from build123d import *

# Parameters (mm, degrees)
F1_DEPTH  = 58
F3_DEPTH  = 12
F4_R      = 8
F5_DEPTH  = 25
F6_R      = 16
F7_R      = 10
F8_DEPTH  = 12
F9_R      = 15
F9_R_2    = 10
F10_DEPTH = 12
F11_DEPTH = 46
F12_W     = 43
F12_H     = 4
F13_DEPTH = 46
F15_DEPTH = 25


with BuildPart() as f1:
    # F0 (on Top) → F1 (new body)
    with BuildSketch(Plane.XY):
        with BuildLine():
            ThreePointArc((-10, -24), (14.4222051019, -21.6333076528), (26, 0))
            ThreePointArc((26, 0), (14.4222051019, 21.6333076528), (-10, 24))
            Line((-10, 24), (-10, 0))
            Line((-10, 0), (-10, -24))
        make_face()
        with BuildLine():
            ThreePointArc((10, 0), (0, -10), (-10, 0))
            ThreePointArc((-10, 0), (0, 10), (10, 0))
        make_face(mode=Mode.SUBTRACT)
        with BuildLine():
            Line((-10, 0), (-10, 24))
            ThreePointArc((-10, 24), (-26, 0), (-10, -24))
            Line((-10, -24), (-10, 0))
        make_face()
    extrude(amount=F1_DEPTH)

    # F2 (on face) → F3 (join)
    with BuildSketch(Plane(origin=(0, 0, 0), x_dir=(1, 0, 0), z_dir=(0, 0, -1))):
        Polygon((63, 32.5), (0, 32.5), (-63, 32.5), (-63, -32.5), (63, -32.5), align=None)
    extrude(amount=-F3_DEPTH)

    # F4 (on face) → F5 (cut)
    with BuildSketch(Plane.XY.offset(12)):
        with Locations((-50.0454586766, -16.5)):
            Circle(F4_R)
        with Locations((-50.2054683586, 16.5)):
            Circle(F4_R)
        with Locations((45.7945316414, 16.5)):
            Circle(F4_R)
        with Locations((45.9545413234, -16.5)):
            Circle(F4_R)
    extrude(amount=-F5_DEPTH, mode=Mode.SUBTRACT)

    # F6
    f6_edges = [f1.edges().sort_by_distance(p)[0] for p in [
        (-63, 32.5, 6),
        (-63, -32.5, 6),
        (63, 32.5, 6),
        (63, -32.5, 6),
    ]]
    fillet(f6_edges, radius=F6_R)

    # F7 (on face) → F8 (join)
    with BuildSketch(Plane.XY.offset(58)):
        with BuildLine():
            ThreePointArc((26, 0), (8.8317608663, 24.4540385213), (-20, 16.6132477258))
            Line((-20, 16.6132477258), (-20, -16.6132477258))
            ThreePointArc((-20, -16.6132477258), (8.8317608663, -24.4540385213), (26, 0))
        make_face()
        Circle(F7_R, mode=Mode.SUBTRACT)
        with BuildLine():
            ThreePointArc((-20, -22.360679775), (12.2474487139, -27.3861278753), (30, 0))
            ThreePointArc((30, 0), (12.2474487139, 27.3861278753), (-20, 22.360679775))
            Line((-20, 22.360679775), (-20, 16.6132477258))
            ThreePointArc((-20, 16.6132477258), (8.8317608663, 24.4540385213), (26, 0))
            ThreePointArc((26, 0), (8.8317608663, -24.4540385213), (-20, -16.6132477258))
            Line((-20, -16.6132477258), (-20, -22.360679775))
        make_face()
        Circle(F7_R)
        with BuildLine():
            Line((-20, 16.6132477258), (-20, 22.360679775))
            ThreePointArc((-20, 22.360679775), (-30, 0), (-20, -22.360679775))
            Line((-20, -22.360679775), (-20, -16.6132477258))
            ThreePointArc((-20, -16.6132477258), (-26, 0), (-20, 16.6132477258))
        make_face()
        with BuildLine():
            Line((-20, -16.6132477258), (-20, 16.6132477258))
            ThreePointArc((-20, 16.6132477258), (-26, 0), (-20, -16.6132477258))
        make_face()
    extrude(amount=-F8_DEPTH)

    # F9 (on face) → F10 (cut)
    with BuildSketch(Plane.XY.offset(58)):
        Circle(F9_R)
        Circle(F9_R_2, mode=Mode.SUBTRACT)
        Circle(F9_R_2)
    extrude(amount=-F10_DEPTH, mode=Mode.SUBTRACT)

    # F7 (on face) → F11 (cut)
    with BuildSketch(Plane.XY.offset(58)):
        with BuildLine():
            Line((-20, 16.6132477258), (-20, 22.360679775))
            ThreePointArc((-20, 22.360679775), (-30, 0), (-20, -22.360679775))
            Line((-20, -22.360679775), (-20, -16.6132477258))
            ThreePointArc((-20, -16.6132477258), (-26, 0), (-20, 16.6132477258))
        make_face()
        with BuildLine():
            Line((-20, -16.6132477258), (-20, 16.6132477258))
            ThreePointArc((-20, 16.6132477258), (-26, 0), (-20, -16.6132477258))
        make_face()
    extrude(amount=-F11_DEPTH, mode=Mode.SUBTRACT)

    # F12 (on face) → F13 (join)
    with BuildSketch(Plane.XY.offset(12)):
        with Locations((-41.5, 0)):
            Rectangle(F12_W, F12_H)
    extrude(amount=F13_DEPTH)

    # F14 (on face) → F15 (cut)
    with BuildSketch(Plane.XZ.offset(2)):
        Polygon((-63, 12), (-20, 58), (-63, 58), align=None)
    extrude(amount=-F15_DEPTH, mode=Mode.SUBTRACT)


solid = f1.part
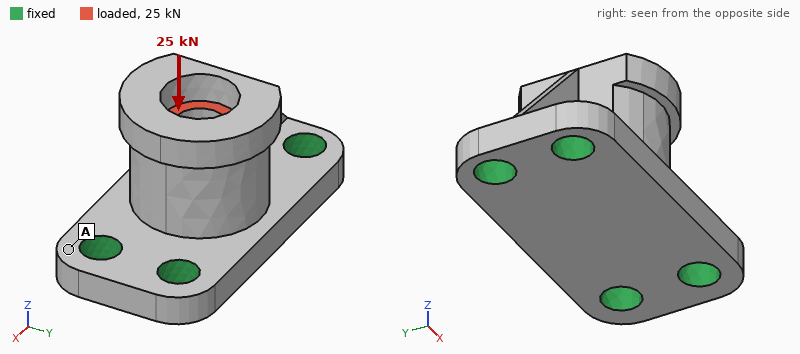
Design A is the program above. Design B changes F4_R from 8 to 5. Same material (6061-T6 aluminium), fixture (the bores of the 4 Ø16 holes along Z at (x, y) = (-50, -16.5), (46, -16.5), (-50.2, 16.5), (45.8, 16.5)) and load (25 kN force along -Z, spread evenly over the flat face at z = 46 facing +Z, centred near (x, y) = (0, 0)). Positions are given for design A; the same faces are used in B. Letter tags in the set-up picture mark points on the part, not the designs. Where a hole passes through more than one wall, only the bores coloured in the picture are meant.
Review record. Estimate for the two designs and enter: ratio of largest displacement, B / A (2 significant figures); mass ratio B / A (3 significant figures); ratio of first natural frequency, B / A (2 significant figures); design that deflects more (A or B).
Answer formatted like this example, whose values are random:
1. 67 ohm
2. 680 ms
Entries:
1. 1.3
2. 1.03
3. 0.89
4. B
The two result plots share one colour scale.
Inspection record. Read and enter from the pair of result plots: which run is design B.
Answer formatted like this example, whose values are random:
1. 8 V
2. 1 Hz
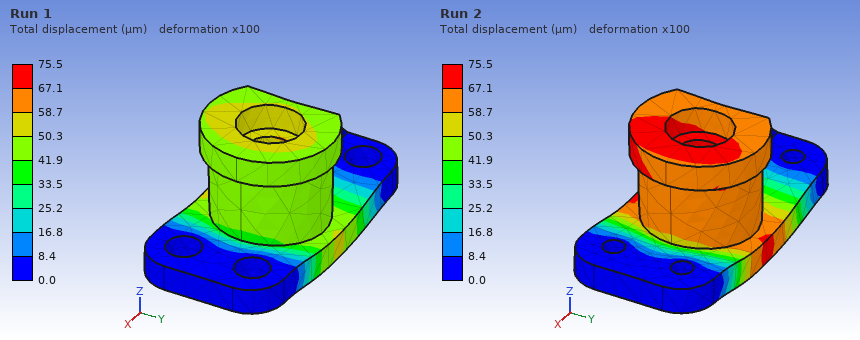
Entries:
1. Run 2
